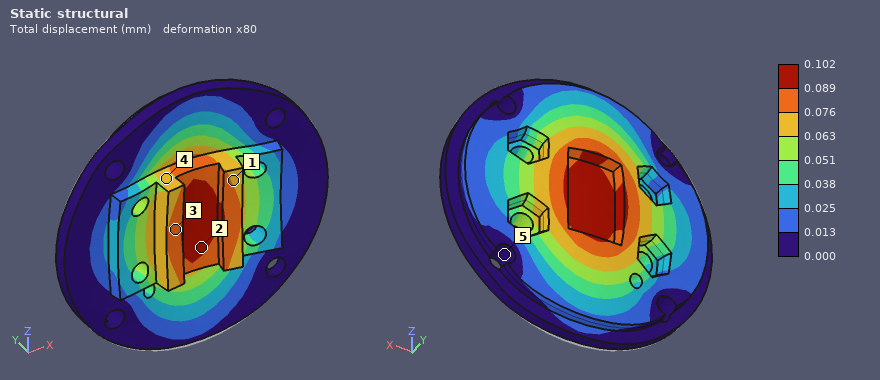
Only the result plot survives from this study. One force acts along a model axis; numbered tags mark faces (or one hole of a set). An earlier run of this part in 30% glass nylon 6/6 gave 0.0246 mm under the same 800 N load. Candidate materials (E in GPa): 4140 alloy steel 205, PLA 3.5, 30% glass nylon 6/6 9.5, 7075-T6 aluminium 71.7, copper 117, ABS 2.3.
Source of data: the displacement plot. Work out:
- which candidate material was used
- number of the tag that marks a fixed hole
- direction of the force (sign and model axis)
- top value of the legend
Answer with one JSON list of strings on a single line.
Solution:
["ABS", "5", "+Y", "0.102 mm"]
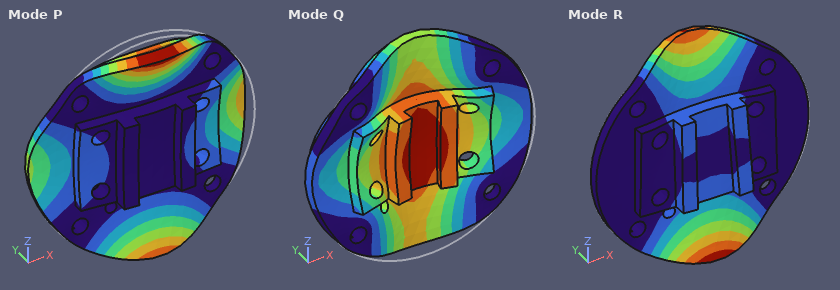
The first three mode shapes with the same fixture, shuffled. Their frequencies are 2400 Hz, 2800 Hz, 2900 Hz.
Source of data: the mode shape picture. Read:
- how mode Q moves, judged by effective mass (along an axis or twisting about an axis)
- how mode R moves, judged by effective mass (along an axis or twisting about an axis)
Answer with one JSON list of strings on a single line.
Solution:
["along Y", "twisting about X"]
